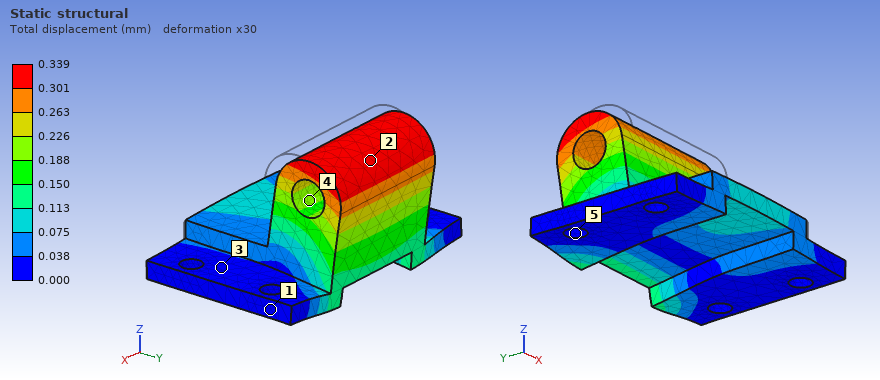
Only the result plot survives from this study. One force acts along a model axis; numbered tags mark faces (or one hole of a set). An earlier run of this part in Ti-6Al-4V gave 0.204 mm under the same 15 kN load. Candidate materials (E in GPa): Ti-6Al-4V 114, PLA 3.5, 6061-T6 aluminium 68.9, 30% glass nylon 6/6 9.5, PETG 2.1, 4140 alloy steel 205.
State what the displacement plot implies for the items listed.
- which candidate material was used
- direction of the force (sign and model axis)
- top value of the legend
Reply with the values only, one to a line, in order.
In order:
6061-T6 aluminium
+Y
0.339 mm
